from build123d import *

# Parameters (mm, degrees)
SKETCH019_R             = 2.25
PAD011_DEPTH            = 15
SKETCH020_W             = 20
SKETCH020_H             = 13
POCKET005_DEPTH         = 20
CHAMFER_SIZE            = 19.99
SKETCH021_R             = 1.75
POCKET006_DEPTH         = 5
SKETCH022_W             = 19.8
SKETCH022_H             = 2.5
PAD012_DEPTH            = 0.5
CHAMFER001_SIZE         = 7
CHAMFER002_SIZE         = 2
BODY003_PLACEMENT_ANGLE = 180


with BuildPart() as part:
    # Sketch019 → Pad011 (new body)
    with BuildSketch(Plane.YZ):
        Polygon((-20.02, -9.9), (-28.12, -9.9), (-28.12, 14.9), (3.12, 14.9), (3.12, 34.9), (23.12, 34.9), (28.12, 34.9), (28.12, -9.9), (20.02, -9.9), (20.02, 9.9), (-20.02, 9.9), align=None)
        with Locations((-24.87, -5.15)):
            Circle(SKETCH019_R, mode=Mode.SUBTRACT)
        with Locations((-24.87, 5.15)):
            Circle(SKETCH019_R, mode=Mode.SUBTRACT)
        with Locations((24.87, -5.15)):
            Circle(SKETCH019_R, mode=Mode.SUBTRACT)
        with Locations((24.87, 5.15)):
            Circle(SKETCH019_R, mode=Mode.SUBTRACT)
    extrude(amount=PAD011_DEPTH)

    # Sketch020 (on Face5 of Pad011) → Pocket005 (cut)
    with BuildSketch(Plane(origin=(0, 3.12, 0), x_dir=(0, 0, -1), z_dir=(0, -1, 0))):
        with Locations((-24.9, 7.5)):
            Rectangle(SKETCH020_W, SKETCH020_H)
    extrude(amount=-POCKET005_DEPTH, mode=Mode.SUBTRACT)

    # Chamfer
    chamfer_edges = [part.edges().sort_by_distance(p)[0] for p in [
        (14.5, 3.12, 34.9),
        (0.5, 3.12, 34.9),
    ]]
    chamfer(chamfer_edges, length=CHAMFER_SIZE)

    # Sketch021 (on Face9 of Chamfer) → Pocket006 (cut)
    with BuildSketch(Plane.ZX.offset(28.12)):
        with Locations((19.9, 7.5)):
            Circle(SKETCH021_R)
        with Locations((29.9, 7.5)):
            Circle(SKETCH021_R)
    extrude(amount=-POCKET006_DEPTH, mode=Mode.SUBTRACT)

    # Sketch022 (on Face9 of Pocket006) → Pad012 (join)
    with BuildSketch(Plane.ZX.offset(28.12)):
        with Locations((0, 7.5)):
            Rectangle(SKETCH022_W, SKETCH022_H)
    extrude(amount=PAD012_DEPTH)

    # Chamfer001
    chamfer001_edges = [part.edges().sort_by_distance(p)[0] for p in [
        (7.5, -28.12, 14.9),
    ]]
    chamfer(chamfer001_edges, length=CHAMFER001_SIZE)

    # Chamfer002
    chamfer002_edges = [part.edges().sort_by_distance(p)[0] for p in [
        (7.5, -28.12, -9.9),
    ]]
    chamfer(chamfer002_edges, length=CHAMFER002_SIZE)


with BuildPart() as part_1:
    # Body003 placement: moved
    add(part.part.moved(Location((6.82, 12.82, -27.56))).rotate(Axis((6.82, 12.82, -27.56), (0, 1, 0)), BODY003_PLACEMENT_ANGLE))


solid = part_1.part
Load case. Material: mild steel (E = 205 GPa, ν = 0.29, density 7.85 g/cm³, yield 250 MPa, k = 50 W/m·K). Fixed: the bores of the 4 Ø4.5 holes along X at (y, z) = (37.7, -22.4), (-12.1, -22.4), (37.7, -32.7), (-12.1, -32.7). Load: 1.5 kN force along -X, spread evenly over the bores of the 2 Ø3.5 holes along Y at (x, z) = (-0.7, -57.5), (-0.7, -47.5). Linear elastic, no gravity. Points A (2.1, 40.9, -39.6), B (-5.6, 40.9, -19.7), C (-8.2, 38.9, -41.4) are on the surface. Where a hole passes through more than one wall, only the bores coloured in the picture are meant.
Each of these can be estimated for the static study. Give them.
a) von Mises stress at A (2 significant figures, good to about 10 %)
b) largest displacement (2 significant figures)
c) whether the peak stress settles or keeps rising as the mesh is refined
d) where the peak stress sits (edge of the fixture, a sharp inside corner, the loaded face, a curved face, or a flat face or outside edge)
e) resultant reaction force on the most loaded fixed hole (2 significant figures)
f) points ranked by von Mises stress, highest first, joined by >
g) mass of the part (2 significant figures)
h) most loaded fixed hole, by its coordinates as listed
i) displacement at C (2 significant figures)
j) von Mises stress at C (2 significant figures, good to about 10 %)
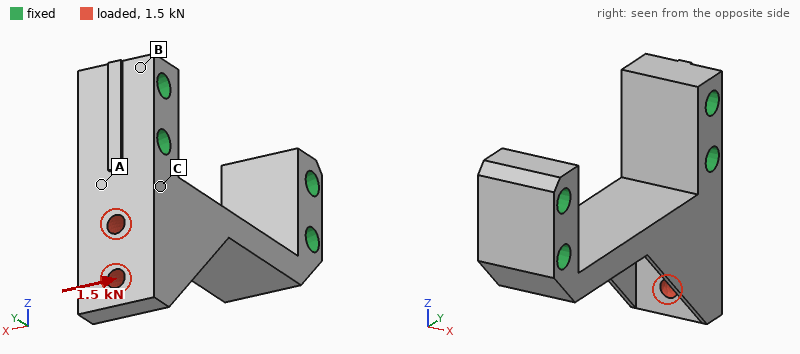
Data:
43 MPa
21 µm
keeps rising
edge of the fixture
1.6 kN
C > A > B
75 g
(37.7, -32.7)
4.4 µm
75 MPa
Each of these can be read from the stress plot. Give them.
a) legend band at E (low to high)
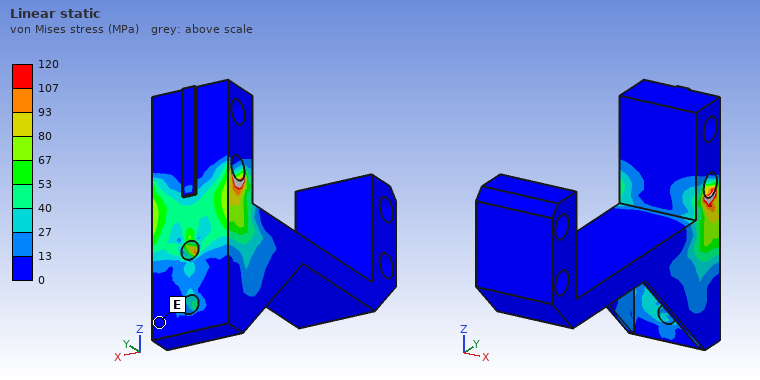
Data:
0 to 13 MPa
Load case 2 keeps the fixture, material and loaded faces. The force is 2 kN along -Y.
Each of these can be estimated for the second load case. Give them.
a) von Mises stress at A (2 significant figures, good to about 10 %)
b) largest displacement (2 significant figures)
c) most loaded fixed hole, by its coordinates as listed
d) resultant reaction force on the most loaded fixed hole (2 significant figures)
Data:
85 MPa
40 µm
(-12.1, -32.7)
1.5 kN
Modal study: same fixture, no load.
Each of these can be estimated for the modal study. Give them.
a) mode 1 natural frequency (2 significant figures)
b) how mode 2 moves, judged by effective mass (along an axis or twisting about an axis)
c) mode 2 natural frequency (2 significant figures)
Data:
9600 Hz
along X
13 kHz
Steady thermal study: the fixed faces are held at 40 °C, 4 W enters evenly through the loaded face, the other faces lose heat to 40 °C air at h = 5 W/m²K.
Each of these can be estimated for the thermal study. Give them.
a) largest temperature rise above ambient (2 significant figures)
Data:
16 K
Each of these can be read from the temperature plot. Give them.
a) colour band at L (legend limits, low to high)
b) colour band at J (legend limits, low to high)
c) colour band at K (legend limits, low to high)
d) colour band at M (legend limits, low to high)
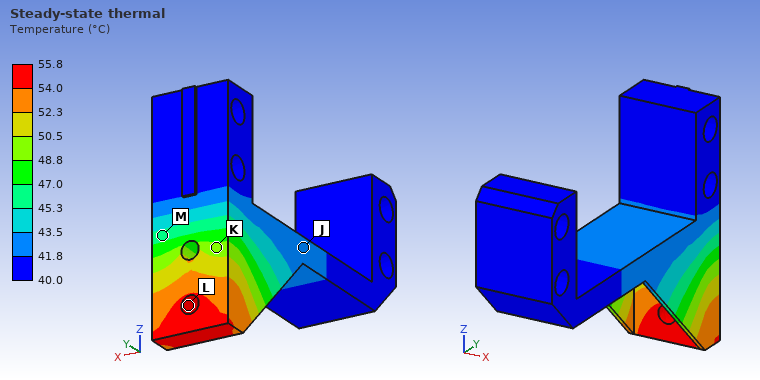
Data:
54.0 to 55.8 °C
41.8 to 43.5 °C
48.8 to 50.5 °C
45.3 to 47.0 °C
